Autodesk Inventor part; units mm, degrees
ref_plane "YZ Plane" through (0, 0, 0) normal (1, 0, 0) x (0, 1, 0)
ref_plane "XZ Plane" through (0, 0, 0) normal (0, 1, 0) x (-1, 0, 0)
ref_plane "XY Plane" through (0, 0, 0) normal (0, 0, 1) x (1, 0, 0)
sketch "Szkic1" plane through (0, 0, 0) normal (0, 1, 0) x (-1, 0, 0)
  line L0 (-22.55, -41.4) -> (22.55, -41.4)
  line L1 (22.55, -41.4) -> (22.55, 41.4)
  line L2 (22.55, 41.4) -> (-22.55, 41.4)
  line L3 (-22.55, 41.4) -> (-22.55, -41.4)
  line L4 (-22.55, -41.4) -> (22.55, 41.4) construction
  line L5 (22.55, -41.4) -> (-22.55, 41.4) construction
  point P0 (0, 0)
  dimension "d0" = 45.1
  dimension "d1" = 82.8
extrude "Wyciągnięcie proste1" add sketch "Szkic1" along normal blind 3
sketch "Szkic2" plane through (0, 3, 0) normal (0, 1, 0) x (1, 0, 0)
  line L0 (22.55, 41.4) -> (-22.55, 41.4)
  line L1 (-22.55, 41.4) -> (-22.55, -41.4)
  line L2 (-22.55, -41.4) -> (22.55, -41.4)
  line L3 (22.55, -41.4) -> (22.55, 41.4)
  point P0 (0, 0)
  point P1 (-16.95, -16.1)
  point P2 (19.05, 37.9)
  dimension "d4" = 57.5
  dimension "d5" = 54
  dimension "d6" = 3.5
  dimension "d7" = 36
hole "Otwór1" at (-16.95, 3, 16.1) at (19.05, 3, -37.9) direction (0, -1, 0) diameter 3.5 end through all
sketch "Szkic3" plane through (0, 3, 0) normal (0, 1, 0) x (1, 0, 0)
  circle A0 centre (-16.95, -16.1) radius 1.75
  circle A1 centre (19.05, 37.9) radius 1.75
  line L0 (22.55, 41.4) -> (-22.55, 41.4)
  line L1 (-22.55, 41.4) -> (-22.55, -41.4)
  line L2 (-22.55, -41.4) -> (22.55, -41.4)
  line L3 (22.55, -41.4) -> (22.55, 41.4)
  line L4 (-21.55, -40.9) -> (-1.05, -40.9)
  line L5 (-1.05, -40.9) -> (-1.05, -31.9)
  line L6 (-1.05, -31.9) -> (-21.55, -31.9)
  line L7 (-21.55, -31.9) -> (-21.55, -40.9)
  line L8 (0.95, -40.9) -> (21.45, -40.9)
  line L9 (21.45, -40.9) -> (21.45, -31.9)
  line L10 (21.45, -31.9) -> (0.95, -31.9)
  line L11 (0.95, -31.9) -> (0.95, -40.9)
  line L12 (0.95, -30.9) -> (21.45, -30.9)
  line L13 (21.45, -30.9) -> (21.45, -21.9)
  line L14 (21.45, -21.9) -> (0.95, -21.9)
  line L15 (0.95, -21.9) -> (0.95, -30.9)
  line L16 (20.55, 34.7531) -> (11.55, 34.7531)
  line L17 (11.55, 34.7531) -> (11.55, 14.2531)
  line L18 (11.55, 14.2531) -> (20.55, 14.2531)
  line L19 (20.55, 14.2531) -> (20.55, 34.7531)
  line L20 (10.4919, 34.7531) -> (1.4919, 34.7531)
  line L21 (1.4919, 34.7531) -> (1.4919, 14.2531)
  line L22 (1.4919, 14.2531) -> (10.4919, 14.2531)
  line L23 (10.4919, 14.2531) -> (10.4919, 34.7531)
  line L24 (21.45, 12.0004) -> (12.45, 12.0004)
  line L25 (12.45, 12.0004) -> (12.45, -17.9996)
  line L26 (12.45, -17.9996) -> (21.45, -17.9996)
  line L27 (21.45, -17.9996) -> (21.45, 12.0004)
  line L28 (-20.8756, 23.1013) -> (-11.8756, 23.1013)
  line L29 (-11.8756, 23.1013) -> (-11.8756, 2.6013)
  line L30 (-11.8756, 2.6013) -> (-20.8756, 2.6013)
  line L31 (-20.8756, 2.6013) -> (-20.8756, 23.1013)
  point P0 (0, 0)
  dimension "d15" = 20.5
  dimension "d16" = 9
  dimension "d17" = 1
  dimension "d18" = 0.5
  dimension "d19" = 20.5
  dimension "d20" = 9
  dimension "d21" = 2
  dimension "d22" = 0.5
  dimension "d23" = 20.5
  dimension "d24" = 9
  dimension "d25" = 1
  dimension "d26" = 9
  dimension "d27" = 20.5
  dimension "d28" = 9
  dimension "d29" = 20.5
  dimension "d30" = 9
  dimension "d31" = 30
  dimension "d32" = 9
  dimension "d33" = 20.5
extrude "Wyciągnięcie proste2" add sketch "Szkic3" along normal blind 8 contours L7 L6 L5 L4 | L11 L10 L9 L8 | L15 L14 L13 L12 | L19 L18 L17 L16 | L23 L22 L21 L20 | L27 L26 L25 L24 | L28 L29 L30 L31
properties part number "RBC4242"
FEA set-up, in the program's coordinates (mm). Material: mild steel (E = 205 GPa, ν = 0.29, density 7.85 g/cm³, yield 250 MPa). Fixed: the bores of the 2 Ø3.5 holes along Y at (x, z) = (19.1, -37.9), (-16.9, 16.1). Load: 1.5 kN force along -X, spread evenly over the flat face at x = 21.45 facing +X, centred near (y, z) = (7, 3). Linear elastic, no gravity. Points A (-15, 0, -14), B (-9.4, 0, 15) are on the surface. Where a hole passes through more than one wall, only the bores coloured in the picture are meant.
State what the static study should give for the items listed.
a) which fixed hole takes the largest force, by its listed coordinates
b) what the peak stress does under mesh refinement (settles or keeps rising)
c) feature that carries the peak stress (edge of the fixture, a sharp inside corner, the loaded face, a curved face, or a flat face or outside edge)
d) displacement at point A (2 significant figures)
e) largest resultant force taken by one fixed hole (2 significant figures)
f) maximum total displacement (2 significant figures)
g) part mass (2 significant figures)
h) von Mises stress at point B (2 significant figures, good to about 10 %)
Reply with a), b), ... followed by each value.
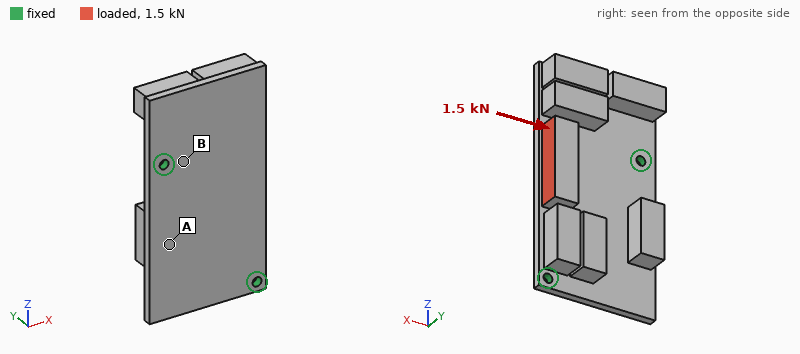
a) (-16.9, 16.1)
b) keeps rising
c) edge of the fixture
d) 0.029 mm
e) 1.0 kN
f) 0.11 mm
g) 170 g
h) 35 MPa
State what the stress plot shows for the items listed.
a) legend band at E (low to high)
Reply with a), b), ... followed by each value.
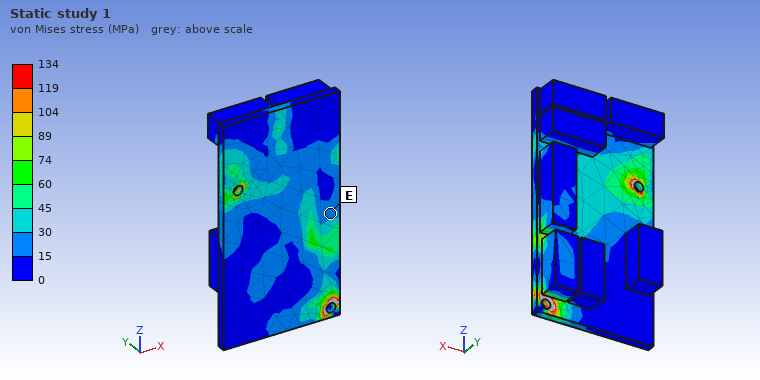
a) 15 to 30 MPa
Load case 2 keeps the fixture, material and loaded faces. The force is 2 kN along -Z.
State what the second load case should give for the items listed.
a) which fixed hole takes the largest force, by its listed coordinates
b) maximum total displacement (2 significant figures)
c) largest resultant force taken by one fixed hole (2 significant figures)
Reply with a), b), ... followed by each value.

a) (19.1, -37.9)
b) 0.12 mm
c) 1.5 kN
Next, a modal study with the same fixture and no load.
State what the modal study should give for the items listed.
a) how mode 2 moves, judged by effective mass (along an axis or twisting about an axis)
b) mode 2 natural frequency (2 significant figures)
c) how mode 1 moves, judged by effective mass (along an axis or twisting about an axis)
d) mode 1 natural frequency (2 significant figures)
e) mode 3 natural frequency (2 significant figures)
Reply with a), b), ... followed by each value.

a) along Y
b) 2200 Hz
c) along Y
d) 1000 Hz
e) 2500 Hz
